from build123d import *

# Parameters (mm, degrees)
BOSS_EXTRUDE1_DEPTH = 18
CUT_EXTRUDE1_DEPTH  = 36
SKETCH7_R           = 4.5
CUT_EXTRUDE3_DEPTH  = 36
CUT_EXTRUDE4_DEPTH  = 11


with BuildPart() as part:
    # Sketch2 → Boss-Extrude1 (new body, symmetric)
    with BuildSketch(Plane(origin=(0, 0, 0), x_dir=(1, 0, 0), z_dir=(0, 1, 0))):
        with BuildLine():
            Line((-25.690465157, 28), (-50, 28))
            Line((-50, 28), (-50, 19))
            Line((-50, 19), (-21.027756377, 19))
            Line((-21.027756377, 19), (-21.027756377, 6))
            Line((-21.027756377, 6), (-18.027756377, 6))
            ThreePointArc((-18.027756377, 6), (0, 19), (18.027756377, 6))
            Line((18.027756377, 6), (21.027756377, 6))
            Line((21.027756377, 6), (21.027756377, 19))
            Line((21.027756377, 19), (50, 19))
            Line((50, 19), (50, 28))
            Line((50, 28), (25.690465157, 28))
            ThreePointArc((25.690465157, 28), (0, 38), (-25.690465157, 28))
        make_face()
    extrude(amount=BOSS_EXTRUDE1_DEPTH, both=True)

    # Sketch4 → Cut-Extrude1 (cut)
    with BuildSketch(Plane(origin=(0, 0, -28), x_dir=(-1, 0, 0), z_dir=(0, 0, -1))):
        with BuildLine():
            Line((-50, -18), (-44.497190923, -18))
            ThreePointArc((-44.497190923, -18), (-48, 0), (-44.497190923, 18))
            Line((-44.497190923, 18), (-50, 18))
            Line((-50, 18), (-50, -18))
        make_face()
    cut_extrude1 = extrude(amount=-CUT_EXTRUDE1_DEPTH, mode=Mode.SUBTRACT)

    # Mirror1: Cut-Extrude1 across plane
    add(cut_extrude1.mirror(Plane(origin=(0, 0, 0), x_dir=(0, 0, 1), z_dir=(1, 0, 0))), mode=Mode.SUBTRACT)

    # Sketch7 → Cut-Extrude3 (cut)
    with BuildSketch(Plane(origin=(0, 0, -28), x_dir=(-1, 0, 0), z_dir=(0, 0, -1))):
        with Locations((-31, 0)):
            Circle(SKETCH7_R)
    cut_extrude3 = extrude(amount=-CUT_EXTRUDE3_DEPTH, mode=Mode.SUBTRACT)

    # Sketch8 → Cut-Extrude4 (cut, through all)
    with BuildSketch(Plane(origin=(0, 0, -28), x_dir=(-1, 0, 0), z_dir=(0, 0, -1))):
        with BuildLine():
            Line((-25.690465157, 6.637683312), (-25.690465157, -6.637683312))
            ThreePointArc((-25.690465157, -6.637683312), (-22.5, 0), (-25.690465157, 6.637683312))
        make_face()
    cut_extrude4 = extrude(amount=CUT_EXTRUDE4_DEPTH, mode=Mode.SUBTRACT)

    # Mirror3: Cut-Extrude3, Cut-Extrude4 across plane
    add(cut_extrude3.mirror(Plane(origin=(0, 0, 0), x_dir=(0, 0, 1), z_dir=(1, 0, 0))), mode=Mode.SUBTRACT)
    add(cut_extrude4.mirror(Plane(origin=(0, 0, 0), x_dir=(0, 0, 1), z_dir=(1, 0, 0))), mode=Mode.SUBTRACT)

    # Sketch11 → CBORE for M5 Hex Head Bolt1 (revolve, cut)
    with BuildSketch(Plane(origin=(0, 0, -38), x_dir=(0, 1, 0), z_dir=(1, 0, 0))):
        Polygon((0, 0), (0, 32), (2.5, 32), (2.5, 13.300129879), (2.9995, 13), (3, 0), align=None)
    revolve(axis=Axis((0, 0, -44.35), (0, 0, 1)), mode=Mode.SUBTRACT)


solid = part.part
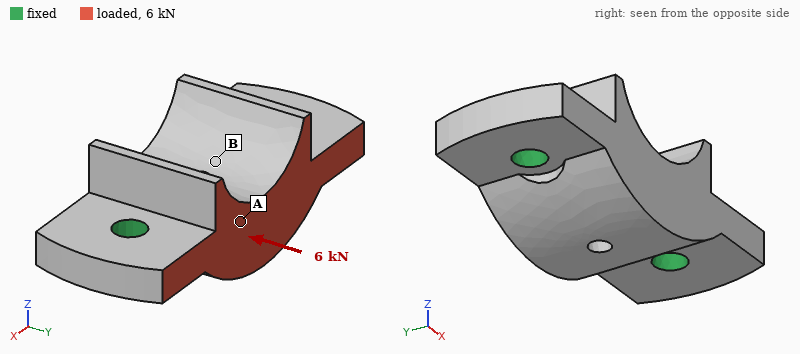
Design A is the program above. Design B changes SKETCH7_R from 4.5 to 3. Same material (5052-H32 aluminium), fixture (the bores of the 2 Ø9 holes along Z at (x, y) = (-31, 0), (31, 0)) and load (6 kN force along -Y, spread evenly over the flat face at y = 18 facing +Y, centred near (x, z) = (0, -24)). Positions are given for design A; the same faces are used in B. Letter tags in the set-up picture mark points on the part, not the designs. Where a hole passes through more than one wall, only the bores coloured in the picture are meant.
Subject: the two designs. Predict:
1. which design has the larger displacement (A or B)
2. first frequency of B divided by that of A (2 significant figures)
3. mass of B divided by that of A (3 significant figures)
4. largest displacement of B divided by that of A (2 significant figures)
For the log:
B
0.83
1.01
1.2
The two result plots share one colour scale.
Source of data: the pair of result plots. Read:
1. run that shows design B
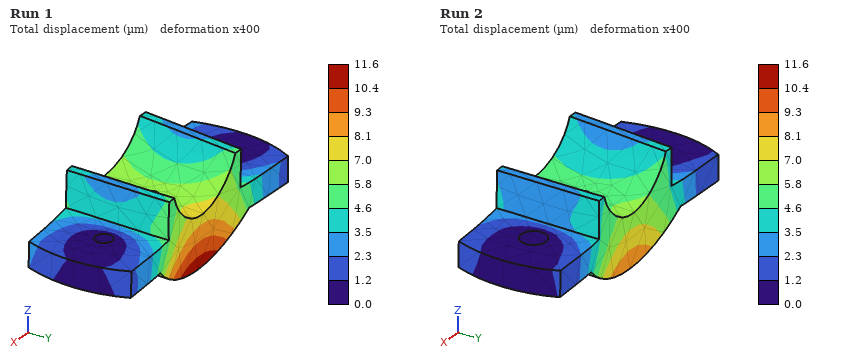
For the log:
Run 1
